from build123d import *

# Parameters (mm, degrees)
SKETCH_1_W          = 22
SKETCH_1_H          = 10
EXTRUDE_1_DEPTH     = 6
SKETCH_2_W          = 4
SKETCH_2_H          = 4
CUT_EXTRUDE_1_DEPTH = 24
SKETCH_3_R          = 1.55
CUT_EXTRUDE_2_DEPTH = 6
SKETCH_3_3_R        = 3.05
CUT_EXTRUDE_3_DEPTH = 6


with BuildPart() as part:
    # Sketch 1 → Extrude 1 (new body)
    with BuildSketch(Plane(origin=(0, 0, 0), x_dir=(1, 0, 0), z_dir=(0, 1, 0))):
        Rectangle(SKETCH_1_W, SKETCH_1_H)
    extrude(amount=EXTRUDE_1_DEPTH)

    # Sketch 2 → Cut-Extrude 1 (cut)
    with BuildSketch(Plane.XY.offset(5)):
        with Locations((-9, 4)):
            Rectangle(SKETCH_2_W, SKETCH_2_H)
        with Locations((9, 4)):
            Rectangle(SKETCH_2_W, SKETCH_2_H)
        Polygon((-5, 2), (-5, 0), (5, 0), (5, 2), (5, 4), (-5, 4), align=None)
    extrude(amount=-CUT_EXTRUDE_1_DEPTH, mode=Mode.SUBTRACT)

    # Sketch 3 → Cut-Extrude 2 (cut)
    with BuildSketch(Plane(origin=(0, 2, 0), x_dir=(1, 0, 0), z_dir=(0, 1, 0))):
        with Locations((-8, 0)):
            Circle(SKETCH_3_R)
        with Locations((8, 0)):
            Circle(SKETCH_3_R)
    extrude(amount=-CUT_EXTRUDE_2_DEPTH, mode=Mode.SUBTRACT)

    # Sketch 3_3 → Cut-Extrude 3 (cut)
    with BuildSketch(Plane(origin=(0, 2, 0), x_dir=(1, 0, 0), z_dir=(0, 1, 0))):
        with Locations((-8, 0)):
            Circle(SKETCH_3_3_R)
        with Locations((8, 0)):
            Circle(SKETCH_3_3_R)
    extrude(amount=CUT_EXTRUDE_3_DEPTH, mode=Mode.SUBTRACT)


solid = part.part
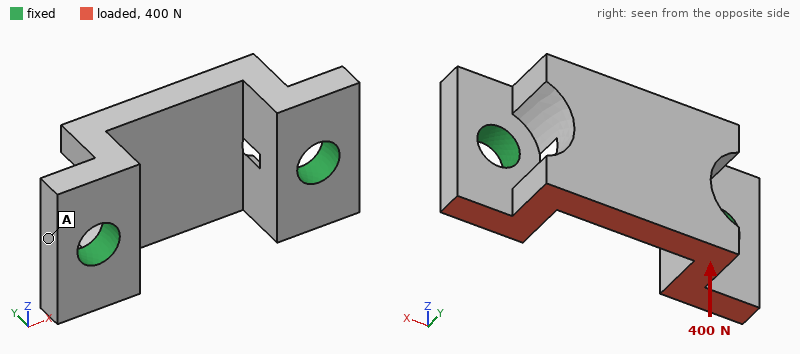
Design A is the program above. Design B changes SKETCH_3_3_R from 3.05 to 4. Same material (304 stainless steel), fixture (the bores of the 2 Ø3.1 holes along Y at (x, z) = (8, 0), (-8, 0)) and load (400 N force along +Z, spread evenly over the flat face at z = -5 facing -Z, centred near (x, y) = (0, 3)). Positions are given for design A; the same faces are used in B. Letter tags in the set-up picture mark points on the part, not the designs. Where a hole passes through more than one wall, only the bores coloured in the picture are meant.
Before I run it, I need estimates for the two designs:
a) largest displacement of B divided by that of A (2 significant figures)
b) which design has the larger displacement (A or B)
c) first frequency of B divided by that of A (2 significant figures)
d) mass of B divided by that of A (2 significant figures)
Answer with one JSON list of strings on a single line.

["1.8", "B", "0.82", "0.89"]
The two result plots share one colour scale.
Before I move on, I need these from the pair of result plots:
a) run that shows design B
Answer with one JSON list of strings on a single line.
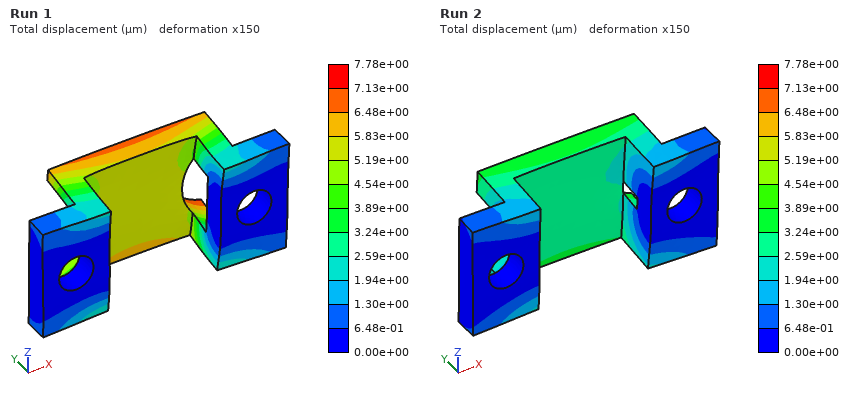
["Run 1"]
